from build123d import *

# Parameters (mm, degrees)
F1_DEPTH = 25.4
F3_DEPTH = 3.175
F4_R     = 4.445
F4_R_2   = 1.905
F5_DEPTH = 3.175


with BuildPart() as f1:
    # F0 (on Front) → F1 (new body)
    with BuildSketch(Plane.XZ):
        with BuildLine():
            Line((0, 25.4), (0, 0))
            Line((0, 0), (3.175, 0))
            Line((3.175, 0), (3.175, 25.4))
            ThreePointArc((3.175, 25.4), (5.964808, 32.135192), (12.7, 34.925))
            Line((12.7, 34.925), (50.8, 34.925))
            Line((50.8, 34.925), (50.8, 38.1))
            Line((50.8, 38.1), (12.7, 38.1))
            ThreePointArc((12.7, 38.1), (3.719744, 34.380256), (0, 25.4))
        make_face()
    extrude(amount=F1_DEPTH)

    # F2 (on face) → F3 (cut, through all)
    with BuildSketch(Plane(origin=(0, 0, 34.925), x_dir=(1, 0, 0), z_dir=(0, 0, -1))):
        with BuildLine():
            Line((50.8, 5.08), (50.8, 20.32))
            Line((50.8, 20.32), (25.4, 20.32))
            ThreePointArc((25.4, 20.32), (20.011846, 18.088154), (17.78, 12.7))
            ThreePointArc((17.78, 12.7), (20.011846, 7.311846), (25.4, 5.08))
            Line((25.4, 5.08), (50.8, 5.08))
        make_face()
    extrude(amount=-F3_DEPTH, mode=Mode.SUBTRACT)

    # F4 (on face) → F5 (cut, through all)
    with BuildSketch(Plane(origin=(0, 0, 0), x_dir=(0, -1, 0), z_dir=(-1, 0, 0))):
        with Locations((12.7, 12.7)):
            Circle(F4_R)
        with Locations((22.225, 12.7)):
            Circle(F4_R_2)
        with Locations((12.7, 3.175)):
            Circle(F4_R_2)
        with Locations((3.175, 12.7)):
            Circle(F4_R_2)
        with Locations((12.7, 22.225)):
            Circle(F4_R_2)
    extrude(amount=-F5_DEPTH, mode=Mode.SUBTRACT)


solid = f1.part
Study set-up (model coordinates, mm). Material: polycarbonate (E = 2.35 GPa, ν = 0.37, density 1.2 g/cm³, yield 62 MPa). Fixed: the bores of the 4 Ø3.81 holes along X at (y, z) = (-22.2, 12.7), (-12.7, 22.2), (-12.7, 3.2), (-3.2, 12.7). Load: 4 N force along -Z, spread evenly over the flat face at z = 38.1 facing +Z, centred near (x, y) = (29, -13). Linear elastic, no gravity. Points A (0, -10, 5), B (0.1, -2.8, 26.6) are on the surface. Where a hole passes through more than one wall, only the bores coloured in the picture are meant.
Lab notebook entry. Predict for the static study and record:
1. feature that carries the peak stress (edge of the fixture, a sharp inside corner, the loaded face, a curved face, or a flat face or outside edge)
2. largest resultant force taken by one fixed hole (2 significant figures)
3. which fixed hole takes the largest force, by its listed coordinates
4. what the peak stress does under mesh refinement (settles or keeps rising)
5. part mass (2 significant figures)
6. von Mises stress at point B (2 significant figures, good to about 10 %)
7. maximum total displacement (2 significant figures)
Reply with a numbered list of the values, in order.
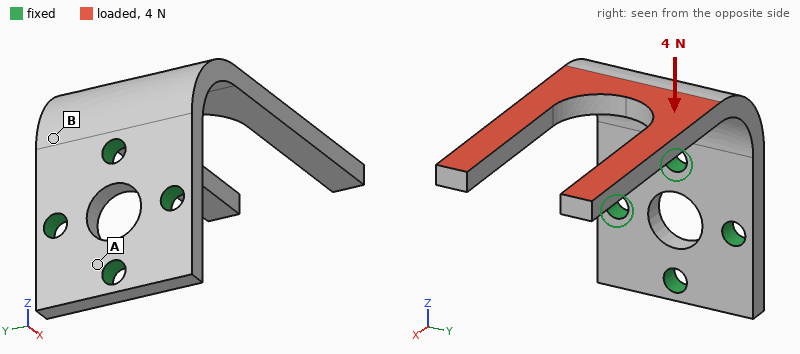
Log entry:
1. edge of the fixture
2. 6.4 N
3. (-12.7, 22.2)
4. keeps rising
5. 5.6 g
6. 1.8 MPa
7. 0.78 mm
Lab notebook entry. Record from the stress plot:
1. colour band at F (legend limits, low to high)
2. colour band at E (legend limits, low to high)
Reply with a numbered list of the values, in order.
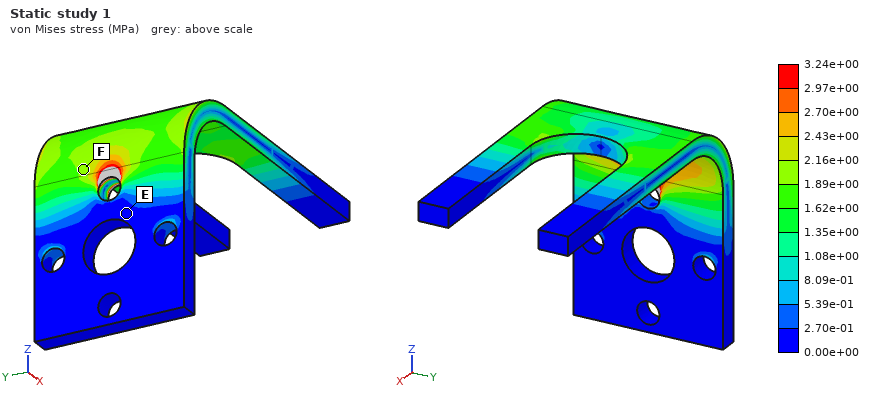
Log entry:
1. 1.89e+00 to 2.16e+00 MPa
2. 0.00e+00 to 2.70e-01 MPa
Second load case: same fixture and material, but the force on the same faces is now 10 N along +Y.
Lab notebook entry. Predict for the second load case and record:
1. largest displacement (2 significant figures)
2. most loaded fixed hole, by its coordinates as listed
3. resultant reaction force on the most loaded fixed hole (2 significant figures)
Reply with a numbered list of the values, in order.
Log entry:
1. 0.71 mm
2. (-12.7, 22.2)
3. 10 N
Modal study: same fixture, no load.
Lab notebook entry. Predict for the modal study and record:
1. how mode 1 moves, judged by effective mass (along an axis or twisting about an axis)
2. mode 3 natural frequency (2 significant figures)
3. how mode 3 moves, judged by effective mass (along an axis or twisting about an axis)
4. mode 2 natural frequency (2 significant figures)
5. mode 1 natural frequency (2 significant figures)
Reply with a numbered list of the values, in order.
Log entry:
1. along Z
2. 560 Hz
3. along Y
4. 470 Hz
5. 330 Hz
